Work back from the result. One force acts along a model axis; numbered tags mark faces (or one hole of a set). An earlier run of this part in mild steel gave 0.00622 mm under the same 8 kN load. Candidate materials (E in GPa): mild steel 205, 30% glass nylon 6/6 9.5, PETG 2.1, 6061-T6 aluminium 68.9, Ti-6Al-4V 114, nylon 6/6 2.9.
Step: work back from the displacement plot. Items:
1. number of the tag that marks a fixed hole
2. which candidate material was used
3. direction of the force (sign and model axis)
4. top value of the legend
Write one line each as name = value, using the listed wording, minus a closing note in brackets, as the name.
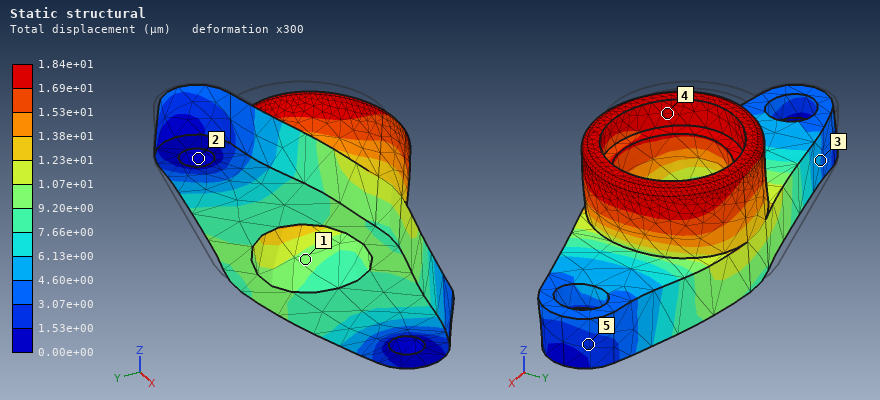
number of the tag that marks a fixed hole = 2
which candidate material was used = 6061-T6 aluminium
direction of the force = +X
top value of the legend = 1.84e+01 µm
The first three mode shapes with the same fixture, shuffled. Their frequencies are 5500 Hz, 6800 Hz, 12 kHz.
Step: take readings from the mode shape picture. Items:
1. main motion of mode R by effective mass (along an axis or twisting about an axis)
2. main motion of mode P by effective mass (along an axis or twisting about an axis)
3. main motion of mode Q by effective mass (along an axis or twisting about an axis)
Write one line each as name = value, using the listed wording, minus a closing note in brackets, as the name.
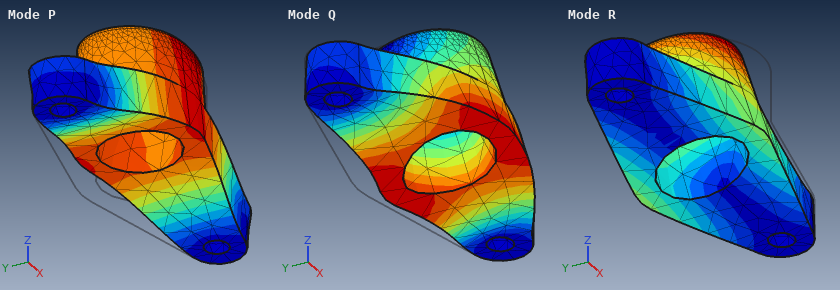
main motion of mode R by effective mass = along Y
main motion of mode P by effective mass = along Z
main motion of mode Q by effective mass = along Y
